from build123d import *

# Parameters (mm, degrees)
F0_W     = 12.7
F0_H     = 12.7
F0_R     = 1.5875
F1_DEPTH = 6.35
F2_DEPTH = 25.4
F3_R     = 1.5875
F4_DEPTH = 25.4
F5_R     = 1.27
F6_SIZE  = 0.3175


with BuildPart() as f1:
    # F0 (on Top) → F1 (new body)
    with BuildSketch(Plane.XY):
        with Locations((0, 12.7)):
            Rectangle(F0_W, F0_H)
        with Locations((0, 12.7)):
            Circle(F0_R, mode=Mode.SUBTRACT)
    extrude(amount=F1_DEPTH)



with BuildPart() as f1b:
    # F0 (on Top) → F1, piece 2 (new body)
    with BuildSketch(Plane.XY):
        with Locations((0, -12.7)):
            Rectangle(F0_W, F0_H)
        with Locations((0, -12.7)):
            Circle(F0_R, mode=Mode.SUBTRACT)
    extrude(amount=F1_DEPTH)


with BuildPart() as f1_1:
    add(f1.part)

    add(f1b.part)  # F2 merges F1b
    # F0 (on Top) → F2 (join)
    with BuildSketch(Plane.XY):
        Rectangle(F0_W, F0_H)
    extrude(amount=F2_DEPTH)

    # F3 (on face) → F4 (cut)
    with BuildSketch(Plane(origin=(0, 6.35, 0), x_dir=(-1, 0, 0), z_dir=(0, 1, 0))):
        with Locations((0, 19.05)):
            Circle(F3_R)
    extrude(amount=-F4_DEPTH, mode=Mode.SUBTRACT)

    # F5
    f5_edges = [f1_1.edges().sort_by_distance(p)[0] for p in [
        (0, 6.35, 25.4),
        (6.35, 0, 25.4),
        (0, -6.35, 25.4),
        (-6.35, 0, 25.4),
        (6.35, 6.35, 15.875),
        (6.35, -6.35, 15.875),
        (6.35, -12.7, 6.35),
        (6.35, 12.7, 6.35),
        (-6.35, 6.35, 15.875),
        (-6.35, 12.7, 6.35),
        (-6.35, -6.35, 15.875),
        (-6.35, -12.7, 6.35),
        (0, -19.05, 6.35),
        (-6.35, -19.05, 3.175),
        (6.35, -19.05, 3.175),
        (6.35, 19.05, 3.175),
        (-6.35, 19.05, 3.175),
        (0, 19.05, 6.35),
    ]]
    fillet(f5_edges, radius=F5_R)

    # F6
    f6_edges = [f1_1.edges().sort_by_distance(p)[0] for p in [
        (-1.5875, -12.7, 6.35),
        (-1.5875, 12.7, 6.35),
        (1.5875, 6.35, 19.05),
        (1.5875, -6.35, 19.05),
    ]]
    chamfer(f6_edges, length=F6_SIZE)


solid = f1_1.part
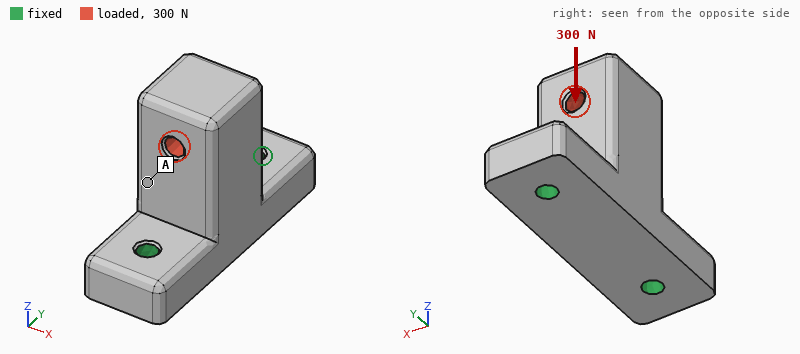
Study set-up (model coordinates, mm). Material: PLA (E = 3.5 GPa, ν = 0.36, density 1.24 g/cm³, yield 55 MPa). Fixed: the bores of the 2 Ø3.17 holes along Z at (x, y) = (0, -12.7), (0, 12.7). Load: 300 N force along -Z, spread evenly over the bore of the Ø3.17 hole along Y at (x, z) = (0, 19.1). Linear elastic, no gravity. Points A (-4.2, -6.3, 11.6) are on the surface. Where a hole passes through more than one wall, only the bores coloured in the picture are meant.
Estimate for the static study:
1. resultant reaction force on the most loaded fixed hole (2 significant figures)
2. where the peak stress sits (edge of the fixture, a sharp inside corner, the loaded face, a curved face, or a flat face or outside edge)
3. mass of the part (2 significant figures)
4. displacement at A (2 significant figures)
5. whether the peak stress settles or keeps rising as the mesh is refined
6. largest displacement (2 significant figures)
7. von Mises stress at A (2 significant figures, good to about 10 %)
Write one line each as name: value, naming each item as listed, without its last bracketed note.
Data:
resultant reaction force on the most loaded fixed hole: 160 N
where the peak stress sits: edge of the fixture
mass of the part: 7.3 g
displacement at A: 27 µm
whether the peak stress settles or keeps rising as the mesh is refined: keeps rising
largest displacement: 34 µm
von Mises stress at A: 1.8 MPa
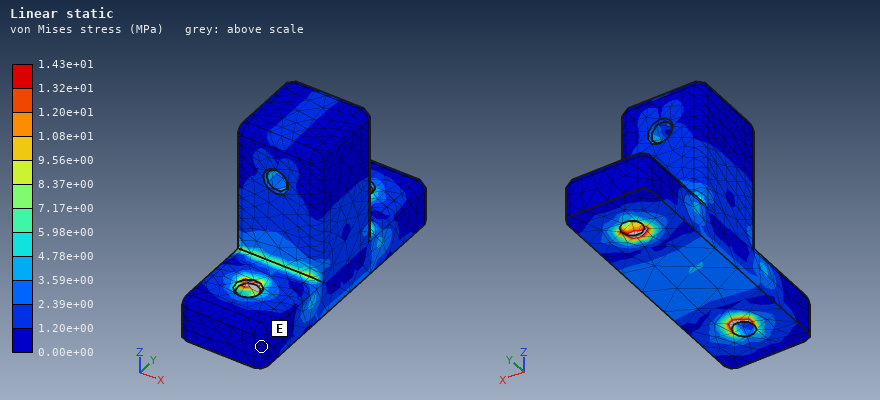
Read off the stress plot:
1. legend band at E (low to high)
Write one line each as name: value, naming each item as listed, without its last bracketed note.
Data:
legend band at E: 0.00e+00 to 1.20e+00 MPa
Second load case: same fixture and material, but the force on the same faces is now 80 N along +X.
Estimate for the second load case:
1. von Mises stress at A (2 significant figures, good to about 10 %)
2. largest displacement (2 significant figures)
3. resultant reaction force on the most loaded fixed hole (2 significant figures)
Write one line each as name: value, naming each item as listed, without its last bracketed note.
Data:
von Mises stress at A: 1.6 MPa
largest displacement: 0.14 mm
resultant reaction force on the most loaded fixed hole: 40 N
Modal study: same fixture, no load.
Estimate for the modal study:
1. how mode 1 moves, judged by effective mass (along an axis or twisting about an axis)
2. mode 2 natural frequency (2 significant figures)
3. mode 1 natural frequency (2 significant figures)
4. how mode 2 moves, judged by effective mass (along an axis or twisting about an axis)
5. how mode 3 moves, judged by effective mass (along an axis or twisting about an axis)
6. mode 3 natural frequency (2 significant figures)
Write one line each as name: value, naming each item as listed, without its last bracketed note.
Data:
how mode 1 moves, judged by effective mass: along X
mode 2 natural frequency: 4800 Hz
mode 1 natural frequency: 2600 Hz
how mode 2 moves, judged by effective mass: along Y
how mode 3 moves, judged by effective mass: along Z
mode 3 natural frequency: 7500 Hz
